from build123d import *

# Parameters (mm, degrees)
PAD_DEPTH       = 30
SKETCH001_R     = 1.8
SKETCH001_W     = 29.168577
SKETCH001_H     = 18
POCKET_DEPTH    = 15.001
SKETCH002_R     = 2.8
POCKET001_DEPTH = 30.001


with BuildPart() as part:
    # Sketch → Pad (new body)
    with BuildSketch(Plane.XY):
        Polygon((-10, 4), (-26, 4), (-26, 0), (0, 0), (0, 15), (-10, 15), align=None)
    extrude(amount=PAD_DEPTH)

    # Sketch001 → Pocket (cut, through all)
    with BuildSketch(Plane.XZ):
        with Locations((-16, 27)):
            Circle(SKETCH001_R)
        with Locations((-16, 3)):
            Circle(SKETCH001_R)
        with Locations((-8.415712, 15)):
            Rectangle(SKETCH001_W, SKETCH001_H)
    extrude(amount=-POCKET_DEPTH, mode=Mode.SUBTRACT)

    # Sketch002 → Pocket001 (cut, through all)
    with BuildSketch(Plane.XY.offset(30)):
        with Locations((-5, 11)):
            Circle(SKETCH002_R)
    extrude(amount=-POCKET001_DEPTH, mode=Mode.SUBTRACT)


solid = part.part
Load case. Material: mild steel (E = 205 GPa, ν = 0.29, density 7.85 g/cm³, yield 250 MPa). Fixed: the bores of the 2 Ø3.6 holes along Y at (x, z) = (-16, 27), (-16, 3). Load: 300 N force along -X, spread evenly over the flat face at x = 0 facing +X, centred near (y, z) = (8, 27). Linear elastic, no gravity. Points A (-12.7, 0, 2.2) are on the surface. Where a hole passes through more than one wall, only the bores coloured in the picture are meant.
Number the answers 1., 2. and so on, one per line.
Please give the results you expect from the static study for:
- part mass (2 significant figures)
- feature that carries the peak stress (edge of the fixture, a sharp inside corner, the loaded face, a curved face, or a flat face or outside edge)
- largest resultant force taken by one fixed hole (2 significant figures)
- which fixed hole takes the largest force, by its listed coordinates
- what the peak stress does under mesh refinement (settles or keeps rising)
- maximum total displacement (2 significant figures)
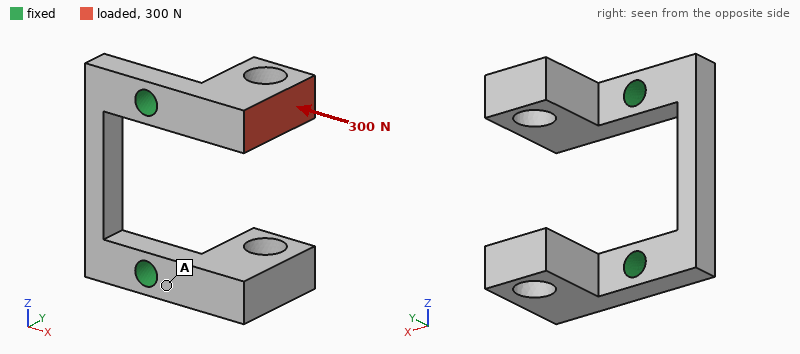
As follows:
1. 19 g
2. edge of the fixture
3. 300 N
4. (-16, 27)
5. keeps rising
6. 31 µm
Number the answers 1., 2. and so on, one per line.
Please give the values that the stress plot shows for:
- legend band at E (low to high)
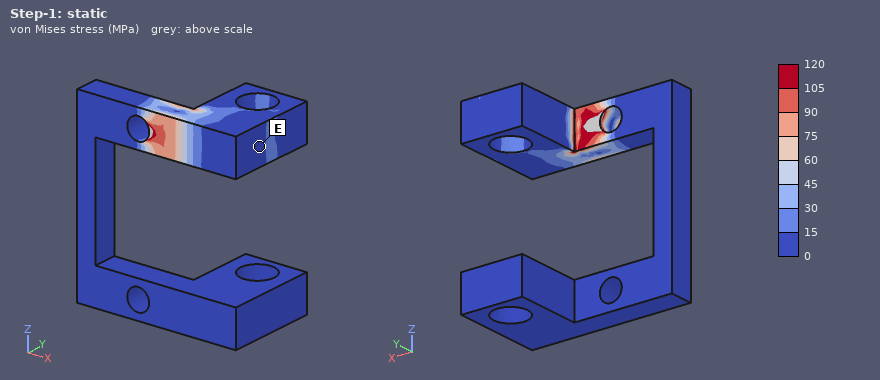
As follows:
1. 0 to 15 MPa
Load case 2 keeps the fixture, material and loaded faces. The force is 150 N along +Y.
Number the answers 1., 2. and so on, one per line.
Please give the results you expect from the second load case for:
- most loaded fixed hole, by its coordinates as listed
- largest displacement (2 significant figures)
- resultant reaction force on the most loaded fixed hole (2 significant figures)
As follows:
1. (-16, 27)
2. 32 µm
3. 150 N
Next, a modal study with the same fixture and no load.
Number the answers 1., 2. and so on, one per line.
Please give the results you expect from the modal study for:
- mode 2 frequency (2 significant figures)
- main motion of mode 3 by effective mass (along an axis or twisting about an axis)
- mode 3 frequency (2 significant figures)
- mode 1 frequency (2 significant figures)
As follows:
1. 6500 Hz
2. along Z
3. 7900 Hz
4. 6500 Hz
